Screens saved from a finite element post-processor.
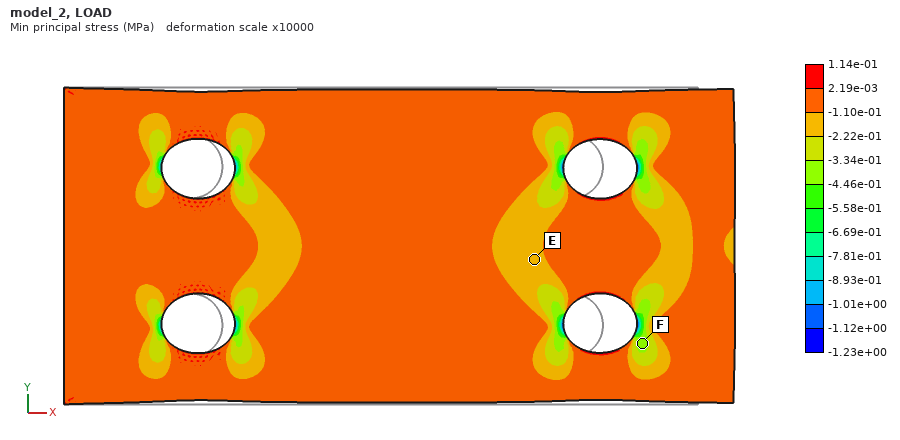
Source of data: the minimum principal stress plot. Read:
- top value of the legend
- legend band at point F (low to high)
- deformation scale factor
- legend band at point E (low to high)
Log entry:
1.14e-01 MPa
-4.46e-01 to -3.34e-01 MPa
10000
-2.22e-01 to -1.10e-01 MPa
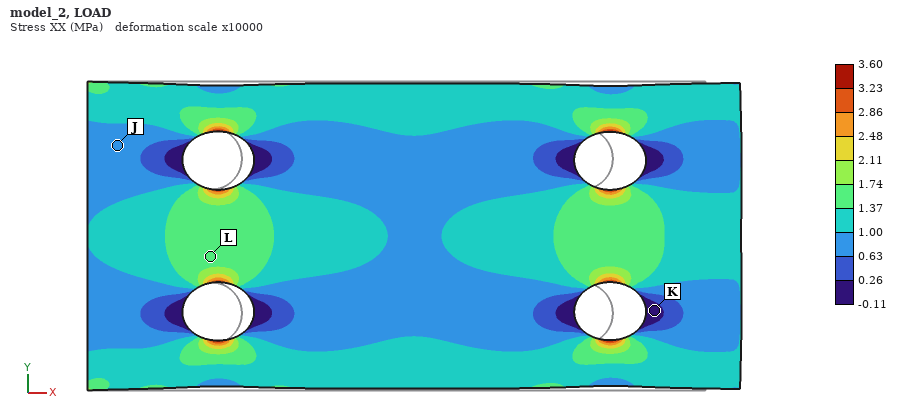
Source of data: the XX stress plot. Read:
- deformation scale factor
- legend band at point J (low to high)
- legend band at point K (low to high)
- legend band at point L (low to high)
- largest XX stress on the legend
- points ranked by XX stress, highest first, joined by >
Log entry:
10000
0.63 to 1.00 MPa
-0.11 to 0.26 MPa
1.37 to 1.74 MPa
3.60 MPa
L > J > K
